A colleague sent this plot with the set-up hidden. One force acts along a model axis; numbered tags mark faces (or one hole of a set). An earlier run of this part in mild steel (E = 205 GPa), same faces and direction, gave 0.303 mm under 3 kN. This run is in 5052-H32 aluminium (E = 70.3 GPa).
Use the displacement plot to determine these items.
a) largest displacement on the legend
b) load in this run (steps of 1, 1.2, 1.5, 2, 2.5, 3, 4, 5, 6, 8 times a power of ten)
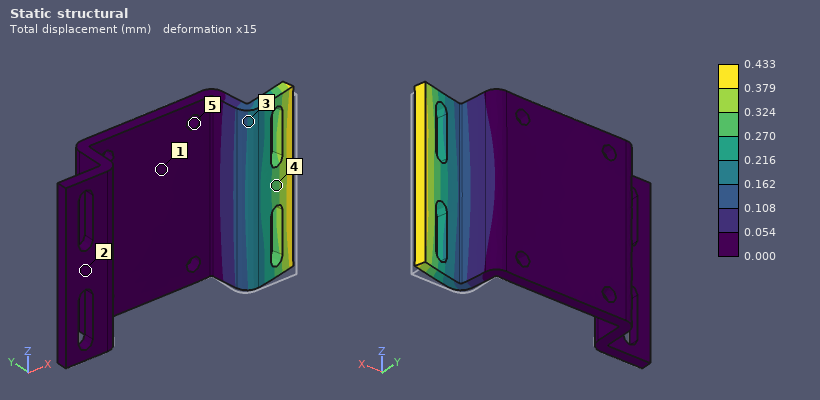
0.433 mm
1.5 kN
